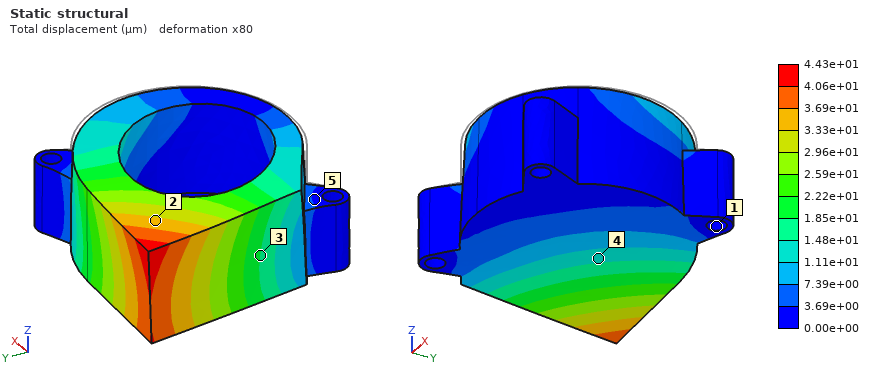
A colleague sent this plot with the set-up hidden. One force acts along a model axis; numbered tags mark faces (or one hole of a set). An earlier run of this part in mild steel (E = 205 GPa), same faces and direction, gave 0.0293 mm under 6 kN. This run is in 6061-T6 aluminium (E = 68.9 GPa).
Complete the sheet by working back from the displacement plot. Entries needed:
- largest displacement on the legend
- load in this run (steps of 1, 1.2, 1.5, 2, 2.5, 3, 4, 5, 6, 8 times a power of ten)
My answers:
4.43e+01 µm
3 kN
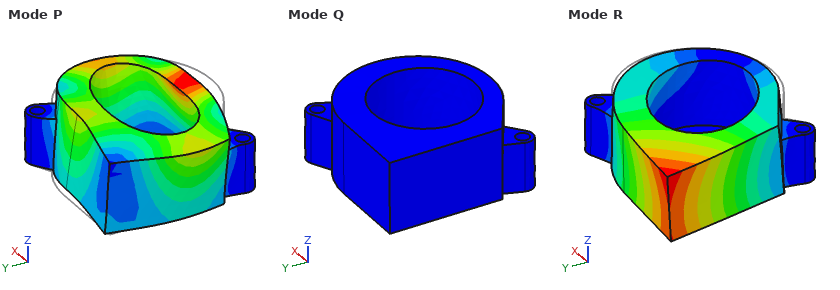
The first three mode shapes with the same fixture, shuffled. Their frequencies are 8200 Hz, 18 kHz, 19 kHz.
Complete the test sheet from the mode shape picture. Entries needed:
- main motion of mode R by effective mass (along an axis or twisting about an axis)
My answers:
along Z
